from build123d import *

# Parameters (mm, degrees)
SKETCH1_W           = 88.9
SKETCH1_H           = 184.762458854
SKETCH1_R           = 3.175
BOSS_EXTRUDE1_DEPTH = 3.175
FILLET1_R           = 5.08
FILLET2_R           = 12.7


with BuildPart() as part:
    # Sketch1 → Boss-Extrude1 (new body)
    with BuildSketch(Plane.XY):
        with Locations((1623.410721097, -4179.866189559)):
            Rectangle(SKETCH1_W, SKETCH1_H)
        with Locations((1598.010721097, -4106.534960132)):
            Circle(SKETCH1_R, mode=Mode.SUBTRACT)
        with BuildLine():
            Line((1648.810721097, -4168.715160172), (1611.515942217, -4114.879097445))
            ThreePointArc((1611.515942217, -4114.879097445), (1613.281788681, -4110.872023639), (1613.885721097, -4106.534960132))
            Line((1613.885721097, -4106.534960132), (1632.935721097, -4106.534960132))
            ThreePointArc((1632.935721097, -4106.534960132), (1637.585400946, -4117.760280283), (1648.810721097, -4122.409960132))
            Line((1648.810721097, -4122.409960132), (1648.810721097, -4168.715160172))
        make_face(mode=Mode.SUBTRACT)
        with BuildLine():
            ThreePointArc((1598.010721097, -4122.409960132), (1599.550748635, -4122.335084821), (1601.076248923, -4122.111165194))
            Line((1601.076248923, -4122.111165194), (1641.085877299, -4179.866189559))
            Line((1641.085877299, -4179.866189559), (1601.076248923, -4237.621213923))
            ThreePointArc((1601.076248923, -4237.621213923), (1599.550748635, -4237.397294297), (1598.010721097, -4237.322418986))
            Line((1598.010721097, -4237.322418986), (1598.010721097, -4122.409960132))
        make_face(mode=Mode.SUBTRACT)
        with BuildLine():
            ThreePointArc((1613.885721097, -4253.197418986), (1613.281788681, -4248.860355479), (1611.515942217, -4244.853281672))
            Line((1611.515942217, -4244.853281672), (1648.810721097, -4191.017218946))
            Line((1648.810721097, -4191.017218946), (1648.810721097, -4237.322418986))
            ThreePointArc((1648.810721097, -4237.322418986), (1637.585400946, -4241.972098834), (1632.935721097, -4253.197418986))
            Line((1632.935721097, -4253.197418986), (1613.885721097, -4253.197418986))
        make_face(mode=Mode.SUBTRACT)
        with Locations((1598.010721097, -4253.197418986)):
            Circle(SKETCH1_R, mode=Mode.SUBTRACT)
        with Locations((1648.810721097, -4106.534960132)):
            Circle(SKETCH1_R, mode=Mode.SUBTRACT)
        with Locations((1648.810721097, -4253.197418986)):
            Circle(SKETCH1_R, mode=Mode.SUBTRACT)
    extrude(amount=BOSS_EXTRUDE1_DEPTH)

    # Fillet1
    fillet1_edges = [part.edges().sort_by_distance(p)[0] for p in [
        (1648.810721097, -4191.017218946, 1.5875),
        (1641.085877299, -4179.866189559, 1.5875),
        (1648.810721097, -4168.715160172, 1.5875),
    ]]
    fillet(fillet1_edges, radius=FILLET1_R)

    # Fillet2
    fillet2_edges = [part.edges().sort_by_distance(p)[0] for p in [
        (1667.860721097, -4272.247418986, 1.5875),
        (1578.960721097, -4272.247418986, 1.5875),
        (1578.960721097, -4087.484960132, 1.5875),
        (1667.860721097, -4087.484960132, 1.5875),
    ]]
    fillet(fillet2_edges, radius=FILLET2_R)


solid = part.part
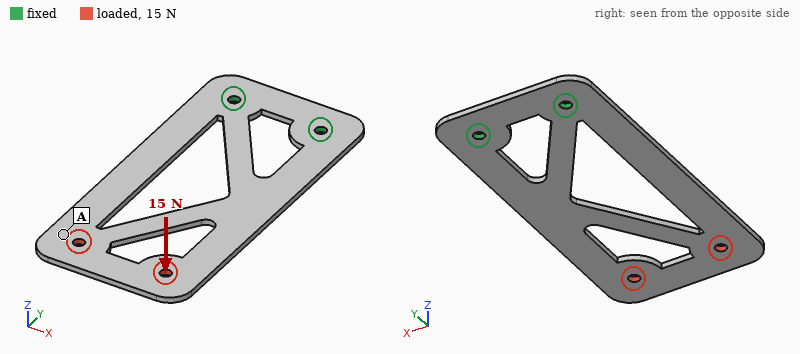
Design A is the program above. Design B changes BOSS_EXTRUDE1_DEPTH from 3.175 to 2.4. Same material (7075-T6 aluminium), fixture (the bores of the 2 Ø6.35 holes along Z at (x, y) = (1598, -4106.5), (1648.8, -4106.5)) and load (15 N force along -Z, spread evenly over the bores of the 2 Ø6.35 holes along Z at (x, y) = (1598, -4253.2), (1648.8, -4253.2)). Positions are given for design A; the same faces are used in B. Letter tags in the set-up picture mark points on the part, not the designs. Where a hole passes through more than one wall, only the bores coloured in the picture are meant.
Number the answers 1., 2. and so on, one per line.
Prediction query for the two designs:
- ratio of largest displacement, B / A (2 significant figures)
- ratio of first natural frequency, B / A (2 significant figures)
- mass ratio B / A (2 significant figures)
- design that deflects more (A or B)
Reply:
1. 2.3
2. 0.76
3. 0.76
4. B
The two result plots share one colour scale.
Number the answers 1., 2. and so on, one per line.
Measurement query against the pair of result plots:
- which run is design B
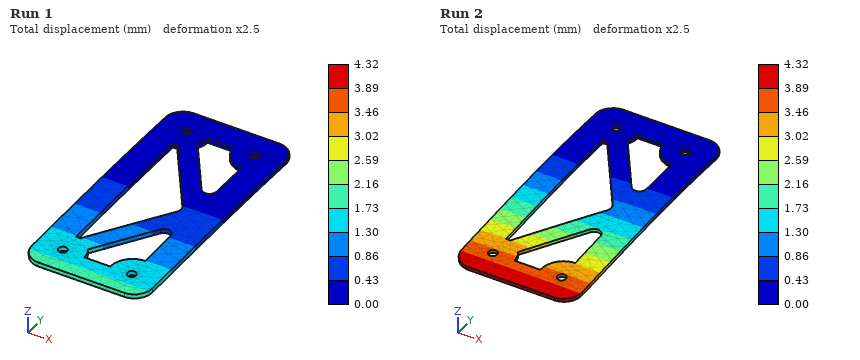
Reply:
1. Run 2
